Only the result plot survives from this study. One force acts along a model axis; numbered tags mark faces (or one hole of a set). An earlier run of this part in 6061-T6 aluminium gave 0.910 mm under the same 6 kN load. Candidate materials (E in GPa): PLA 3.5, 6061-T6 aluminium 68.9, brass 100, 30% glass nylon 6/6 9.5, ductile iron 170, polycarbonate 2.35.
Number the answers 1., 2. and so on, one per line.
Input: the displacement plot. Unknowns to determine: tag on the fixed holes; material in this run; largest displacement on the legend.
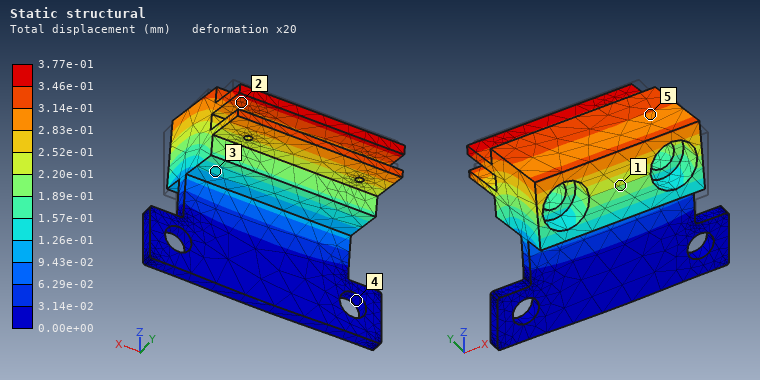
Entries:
1. 4
2. ductile iron
3. 3.77e-01 mm
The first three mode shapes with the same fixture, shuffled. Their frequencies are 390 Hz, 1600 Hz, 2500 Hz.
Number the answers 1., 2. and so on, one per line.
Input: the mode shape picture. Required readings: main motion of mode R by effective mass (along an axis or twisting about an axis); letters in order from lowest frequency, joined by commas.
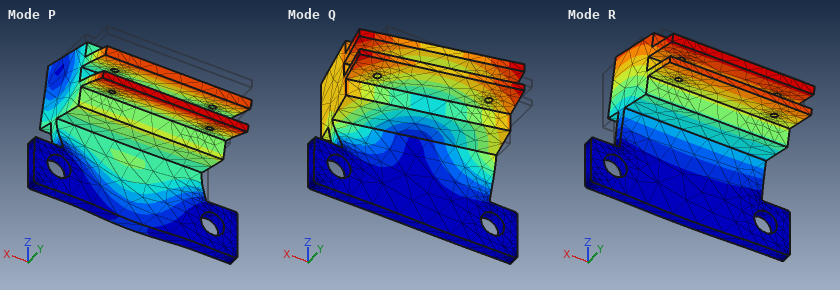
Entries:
1. along Y
2. R, Q, P
